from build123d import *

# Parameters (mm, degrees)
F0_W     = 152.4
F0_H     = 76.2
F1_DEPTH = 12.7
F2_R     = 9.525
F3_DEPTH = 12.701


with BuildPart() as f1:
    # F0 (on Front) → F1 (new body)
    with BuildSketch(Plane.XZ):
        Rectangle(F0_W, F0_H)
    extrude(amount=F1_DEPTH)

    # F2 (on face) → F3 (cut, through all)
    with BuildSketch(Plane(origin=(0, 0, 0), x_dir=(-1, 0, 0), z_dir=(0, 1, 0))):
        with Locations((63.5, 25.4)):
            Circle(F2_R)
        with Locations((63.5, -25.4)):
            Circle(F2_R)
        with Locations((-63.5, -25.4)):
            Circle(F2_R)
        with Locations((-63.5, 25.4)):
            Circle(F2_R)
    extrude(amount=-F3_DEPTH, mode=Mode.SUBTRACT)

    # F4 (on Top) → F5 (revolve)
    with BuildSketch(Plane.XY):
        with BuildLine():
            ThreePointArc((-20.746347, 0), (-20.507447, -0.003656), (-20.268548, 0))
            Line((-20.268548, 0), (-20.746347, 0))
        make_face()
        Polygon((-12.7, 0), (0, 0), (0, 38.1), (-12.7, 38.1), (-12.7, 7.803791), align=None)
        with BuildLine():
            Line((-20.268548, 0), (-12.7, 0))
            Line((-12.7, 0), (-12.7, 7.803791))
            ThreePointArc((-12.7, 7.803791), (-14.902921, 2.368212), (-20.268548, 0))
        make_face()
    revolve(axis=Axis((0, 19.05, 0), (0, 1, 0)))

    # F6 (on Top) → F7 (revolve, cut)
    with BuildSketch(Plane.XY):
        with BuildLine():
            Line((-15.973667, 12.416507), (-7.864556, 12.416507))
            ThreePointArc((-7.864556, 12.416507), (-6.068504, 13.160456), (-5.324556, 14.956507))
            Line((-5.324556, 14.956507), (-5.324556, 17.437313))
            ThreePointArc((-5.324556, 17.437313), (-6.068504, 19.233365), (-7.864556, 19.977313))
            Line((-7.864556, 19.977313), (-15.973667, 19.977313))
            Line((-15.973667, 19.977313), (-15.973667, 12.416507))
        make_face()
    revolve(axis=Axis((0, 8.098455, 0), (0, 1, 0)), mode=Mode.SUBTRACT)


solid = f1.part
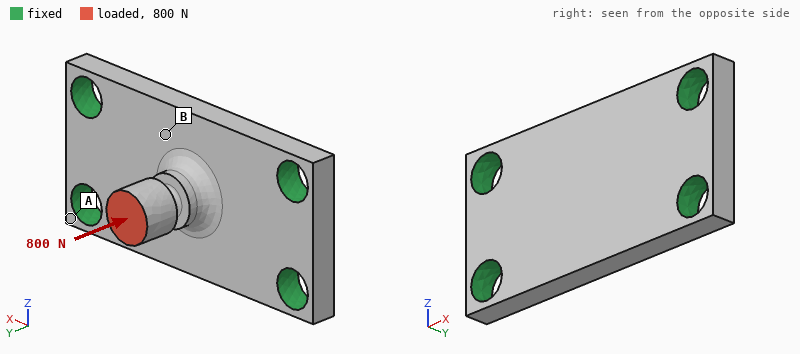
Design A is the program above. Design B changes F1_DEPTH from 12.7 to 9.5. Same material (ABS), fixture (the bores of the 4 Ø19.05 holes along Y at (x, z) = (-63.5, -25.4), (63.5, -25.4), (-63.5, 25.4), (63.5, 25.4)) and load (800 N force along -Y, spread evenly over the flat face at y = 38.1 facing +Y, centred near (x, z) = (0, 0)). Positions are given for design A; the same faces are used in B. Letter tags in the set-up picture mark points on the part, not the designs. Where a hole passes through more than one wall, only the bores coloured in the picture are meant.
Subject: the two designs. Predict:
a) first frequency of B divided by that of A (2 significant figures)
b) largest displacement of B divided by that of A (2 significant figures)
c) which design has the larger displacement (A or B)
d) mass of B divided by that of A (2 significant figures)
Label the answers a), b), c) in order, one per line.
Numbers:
a) 0.87
b) 1.8
c) B
d) 0.78
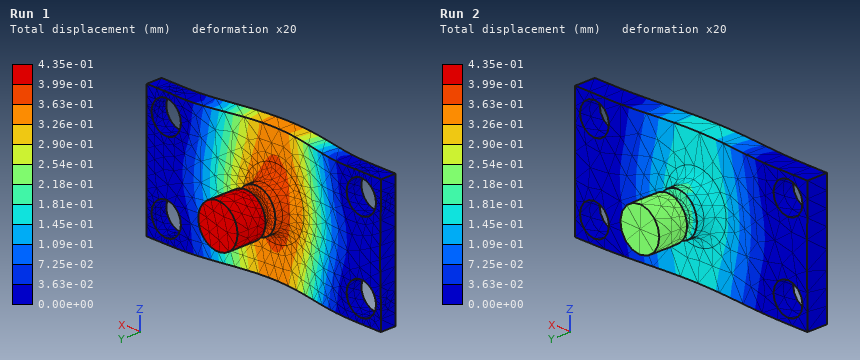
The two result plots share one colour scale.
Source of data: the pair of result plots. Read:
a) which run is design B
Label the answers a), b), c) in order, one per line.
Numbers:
a) Run 1
